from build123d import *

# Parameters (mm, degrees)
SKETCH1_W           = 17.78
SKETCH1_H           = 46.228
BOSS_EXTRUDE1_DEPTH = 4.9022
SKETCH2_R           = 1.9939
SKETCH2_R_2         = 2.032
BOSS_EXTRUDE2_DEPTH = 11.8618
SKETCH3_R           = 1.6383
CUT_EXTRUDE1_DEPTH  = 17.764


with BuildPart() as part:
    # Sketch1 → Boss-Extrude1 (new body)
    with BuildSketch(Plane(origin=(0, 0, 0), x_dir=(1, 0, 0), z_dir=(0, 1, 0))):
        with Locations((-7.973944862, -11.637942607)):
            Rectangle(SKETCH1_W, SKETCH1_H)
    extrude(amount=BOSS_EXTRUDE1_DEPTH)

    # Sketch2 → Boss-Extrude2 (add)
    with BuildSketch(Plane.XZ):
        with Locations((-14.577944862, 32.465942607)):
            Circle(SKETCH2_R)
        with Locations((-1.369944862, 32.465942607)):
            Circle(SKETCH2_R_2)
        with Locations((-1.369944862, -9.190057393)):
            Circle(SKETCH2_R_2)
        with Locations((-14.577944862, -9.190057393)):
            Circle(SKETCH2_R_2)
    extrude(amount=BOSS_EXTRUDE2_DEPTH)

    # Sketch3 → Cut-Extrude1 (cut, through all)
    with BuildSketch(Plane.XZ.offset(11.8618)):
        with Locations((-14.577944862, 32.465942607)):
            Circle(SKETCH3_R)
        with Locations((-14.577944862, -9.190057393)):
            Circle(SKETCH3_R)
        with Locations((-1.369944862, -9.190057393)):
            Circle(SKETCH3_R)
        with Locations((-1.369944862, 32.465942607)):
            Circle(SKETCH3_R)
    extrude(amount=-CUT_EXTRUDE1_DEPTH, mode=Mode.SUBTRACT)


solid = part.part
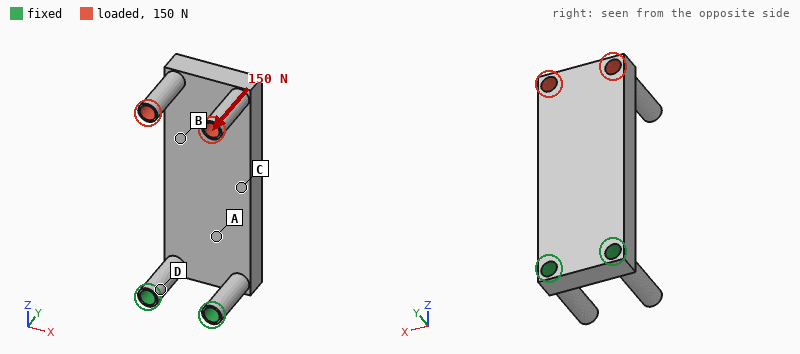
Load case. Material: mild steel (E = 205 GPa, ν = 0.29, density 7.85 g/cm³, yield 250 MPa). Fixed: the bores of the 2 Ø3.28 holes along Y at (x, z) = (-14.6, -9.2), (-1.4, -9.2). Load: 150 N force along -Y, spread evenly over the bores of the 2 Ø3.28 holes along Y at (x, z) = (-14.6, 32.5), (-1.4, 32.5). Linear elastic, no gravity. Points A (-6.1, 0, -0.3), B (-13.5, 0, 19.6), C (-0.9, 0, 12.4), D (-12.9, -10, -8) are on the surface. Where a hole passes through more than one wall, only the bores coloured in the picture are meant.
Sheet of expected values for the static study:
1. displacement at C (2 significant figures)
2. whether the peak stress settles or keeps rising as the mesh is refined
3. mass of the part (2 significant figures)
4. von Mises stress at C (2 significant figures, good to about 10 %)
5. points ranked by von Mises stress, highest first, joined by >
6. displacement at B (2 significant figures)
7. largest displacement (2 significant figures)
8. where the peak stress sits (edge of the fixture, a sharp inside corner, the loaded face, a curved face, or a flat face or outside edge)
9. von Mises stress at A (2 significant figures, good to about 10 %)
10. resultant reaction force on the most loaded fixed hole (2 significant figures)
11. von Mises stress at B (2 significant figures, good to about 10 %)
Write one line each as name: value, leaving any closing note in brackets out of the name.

displacement at C: 0.034 mm
whether the peak stress settles or keeps rising as the mesh is refined: keeps rising
mass of the part: 32 g
von Mises stress at C: 42 MPa
points ranked by von Mises stress, highest first, joined by >: A > C > B > D
displacement at B: 0.056 mm
largest displacement: 0.12 mm
where the peak stress sits: edge of the fixture
von Mises stress at A: 66 MPa
resultant reaction force on the most loaded fixed hole: 75 N
von Mises stress at B: 27 MPa
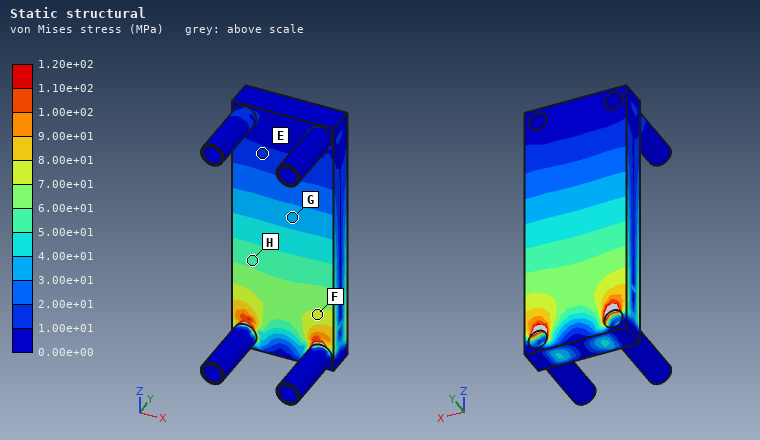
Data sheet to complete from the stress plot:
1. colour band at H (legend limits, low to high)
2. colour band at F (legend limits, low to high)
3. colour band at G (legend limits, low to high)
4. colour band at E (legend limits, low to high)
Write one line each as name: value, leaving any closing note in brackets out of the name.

colour band at H: 5.00e+01 to 6.00e+01 MPa
colour band at F: 7.00e+01 to 8.00e+01 MPa
colour band at G: 3.00e+01 to 4.00e+01 MPa
colour band at E: 1.00e+01 to 2.00e+01 MPa
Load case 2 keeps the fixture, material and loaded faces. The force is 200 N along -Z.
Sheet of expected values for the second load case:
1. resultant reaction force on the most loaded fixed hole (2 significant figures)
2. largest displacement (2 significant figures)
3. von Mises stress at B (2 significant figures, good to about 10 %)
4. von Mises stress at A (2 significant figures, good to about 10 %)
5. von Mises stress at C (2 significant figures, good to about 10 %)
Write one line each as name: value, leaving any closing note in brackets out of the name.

resultant reaction force on the most loaded fixed hole: 100 N
largest displacement: 52 µm
von Mises stress at B: 19 MPa
von Mises stress at A: 18 MPa
von Mises stress at C: 19 MPa
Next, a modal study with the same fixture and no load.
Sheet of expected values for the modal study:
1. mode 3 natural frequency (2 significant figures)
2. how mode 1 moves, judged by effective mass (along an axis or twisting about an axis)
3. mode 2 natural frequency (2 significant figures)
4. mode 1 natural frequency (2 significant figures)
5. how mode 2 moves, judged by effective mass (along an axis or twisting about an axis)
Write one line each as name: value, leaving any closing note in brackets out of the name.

mode 3 natural frequency: 8900 Hz
how mode 1 moves, judged by effective mass: along Y
mode 2 natural frequency: 6900 Hz
mode 1 natural frequency: 2100 Hz
how mode 2 moves, judged by effective mass: along X
